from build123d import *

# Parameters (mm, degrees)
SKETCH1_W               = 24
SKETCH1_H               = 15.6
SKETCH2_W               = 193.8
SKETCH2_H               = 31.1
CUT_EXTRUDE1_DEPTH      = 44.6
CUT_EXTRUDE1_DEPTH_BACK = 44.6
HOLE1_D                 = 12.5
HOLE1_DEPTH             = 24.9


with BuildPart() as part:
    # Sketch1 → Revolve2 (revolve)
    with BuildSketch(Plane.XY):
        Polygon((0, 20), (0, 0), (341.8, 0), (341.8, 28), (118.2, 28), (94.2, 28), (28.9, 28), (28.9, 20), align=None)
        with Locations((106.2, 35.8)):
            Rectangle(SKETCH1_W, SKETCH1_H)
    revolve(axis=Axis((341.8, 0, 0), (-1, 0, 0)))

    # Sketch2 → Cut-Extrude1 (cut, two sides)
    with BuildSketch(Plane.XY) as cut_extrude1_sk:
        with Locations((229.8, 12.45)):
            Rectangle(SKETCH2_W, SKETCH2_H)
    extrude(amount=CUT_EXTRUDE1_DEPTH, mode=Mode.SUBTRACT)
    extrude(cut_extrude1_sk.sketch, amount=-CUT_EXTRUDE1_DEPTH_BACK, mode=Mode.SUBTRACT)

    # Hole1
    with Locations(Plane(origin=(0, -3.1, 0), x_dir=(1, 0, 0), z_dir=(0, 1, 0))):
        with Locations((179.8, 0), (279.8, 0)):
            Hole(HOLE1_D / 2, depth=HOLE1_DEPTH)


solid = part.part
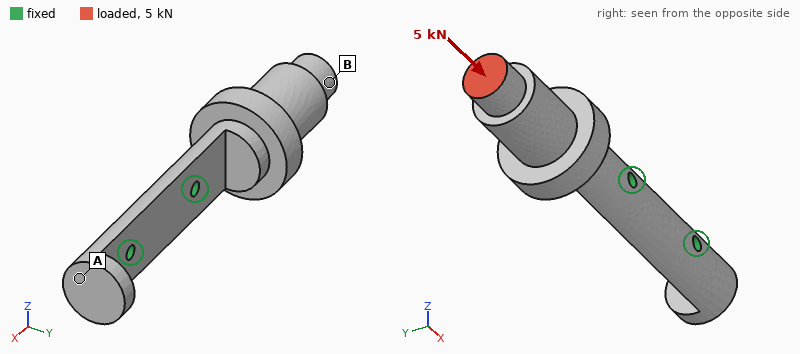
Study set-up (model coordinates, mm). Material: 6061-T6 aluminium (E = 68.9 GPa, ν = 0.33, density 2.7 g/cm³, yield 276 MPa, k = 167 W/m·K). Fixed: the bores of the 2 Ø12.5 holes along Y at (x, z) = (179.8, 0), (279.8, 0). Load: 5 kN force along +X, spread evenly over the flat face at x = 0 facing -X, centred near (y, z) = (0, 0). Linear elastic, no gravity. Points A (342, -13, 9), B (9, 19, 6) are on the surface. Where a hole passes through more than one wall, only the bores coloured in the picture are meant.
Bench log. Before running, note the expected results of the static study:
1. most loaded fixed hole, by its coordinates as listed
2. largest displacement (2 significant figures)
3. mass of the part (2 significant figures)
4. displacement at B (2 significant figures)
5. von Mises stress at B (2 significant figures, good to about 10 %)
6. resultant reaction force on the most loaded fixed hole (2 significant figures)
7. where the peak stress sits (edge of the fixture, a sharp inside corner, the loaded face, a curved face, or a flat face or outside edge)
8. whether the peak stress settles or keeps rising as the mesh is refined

(179.8, 0)
0.19 mm
1.7 kg
0.18 mm
3.9 MPa
4.5 kN
edge of the fixture
keeps rising
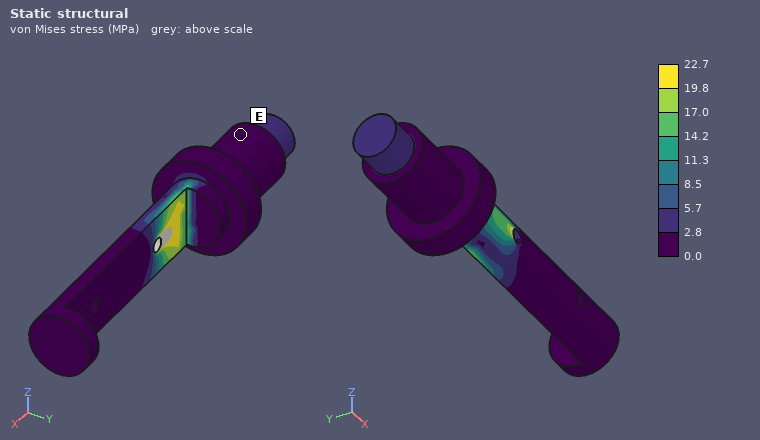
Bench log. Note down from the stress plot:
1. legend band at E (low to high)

0.0 to 2.8 MPa
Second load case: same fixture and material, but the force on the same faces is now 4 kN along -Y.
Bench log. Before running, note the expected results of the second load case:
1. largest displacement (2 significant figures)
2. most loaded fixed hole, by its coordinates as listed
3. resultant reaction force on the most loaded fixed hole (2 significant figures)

1.7 mm
(179.8, 0)
5.2 kN
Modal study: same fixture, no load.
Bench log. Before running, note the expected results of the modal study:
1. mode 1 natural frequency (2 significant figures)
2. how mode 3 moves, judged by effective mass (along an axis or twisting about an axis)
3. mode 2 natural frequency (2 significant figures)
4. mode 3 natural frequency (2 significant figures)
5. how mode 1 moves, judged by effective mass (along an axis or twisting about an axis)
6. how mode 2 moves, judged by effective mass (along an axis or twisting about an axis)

450 Hz
twisting about X
700 Hz
1600 Hz
along Y
along Z
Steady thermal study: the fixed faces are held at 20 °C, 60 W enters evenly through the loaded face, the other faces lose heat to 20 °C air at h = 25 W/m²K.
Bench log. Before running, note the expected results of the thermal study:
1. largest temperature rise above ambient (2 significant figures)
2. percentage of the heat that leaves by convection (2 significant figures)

34 K
28 %
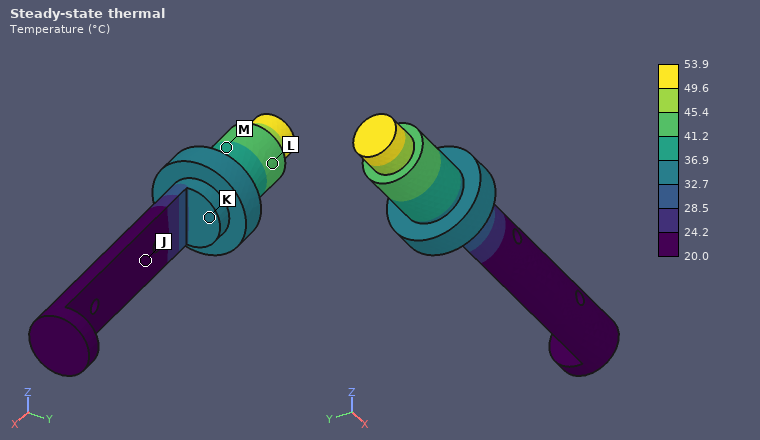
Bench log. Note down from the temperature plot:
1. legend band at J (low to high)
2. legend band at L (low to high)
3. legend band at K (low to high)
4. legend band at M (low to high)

20.0 to 24.2 °C
41.2 to 45.4 °C
32.7 to 36.9 °C
36.9 to 41.2 °C
